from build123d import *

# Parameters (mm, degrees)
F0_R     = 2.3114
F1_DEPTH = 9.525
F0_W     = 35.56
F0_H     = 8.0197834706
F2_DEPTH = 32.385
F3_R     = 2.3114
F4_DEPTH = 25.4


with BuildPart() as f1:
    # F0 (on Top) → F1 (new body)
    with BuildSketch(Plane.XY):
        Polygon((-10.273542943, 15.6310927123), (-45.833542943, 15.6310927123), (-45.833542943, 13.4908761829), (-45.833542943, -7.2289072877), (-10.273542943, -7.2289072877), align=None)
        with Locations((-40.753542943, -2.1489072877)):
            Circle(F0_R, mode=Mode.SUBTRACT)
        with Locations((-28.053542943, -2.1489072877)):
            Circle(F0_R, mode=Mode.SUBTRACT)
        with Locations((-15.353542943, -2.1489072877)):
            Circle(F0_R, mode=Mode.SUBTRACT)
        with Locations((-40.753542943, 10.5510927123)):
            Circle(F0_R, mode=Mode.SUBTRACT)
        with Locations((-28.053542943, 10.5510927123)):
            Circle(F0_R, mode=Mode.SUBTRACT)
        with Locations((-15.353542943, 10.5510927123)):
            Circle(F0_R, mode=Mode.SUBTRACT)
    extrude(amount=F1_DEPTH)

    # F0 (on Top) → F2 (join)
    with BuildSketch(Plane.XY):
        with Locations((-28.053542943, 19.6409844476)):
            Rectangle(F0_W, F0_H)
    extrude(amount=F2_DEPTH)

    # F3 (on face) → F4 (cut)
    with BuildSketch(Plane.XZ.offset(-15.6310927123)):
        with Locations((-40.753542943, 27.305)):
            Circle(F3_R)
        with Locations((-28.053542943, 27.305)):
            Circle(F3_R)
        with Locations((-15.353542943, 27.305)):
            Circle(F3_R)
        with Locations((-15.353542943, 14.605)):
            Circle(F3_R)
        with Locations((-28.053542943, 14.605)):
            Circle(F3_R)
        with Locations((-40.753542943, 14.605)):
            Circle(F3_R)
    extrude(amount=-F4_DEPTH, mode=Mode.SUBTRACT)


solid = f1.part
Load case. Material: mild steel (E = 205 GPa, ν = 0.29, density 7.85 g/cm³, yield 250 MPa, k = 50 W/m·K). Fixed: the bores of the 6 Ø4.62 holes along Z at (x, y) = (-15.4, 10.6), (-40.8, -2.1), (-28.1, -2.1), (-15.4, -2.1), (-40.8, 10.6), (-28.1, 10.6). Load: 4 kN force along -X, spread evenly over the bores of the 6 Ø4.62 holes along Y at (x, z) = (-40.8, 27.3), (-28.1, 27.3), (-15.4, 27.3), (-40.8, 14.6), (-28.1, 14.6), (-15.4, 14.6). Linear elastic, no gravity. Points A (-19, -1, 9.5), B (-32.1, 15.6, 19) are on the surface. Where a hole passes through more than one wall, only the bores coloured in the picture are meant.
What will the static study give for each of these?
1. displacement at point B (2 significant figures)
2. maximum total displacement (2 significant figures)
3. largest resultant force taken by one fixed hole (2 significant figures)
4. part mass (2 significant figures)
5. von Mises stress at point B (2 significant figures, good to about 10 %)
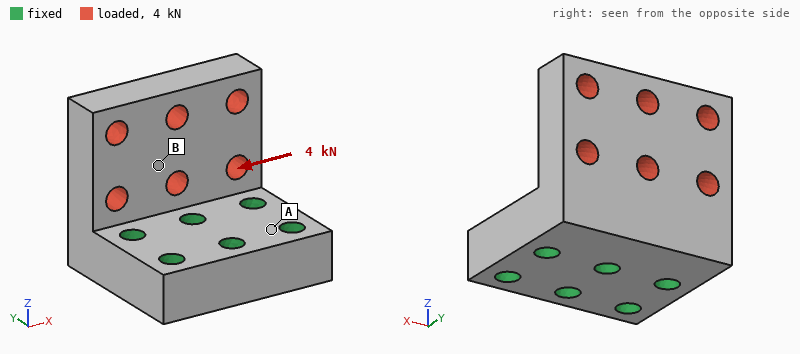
7.7 µm
15 µm
2.6 kN
120 g
21 MPa
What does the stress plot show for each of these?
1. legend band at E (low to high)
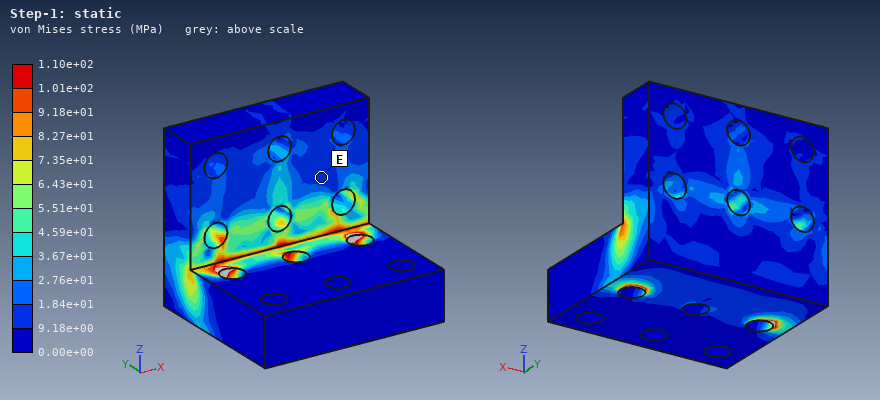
9.18e+00 to 1.84e+01 MPa
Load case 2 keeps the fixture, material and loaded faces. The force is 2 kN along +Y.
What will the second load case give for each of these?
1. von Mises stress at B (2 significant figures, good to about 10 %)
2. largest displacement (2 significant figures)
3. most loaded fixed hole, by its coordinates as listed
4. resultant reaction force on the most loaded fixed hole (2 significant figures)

25 MPa
32 µm
(-28.1, 10.6)
790 N
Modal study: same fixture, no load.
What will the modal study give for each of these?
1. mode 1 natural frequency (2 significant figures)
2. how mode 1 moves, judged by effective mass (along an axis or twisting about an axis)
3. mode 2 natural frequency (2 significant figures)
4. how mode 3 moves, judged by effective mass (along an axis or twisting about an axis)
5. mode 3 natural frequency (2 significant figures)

7200 Hz
along Y
13 kHz
along X
16 kHz
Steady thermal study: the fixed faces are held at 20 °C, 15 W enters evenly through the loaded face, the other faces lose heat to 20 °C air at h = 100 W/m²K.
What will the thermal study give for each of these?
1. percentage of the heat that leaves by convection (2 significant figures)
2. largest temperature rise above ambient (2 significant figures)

23 %
19 K
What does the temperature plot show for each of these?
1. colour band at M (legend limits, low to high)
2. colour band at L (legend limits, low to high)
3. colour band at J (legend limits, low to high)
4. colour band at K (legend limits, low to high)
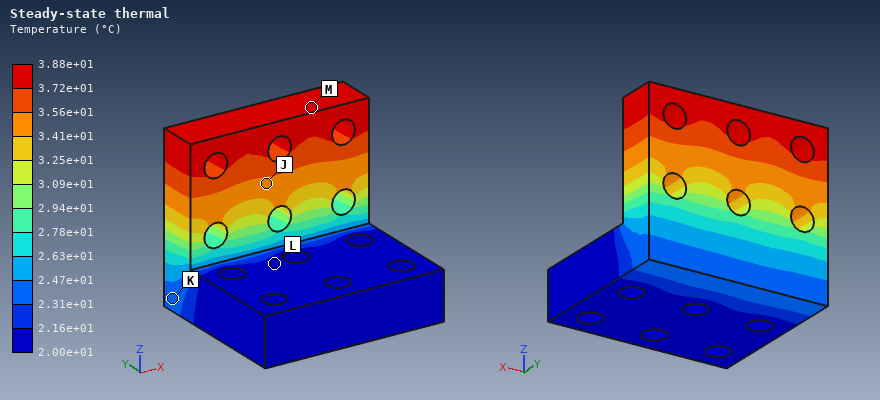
3.72e+01 to 3.88e+01 °C
2.00e+01 to 2.16e+01 °C
3.41e+01 to 3.56e+01 °C
2.31e+01 to 2.47e+01 °C
